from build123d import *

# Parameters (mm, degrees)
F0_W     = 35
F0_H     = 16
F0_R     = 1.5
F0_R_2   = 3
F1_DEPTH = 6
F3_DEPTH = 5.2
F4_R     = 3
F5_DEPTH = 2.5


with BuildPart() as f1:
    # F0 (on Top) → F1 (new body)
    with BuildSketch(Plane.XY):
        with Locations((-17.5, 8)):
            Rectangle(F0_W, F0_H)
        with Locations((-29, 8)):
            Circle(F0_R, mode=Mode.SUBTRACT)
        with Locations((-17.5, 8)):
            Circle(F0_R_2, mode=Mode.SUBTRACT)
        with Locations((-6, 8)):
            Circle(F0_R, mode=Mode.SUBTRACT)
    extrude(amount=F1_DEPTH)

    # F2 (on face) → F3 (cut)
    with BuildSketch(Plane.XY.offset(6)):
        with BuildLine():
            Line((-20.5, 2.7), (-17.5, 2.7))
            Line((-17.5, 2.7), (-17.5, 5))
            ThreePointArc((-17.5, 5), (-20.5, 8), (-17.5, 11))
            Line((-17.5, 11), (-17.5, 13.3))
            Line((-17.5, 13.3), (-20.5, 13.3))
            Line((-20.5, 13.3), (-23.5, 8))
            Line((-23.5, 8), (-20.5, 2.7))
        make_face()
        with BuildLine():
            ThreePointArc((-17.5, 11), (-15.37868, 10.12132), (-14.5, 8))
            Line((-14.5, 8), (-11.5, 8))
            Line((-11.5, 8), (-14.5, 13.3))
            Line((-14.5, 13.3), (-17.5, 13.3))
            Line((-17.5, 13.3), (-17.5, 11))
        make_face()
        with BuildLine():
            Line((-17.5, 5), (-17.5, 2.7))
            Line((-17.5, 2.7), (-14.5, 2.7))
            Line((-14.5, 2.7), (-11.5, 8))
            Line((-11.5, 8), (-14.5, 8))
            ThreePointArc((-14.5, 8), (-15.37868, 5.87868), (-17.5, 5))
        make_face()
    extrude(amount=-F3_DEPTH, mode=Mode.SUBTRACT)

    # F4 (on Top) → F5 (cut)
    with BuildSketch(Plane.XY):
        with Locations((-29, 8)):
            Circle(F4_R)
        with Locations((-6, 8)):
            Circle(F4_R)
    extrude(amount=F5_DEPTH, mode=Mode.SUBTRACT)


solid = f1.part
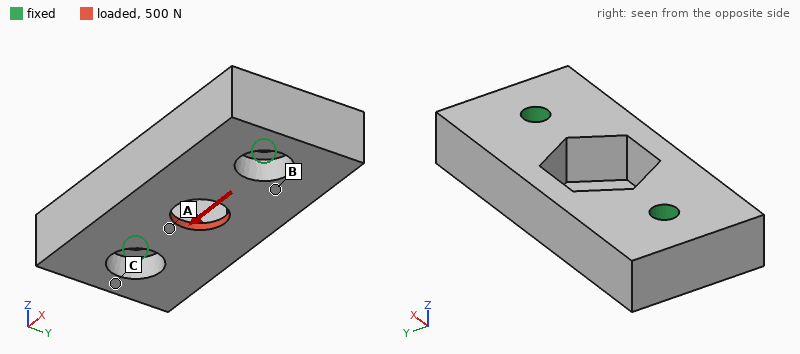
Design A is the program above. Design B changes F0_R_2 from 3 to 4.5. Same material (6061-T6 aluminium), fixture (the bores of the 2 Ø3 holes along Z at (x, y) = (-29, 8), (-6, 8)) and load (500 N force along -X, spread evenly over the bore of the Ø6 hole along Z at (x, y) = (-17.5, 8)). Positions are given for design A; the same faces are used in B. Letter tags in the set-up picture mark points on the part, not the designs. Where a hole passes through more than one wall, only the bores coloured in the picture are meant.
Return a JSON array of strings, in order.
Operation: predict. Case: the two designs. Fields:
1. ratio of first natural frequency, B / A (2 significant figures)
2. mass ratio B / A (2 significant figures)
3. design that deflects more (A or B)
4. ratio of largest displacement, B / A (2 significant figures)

["1.0", "0.99", "A", "0.68"]
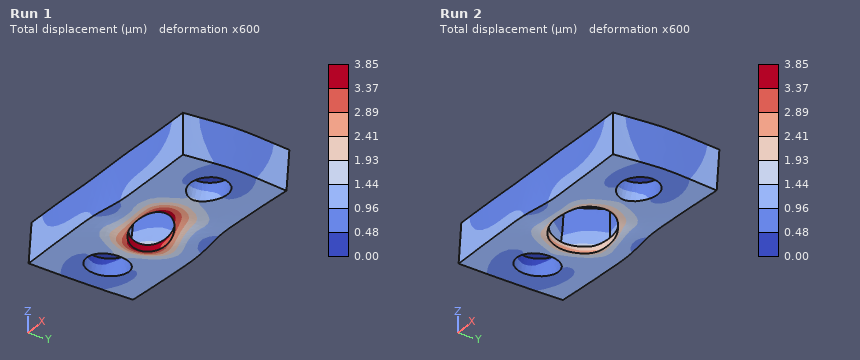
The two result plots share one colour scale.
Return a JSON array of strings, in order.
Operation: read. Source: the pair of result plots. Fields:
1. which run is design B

["Run 2"]
